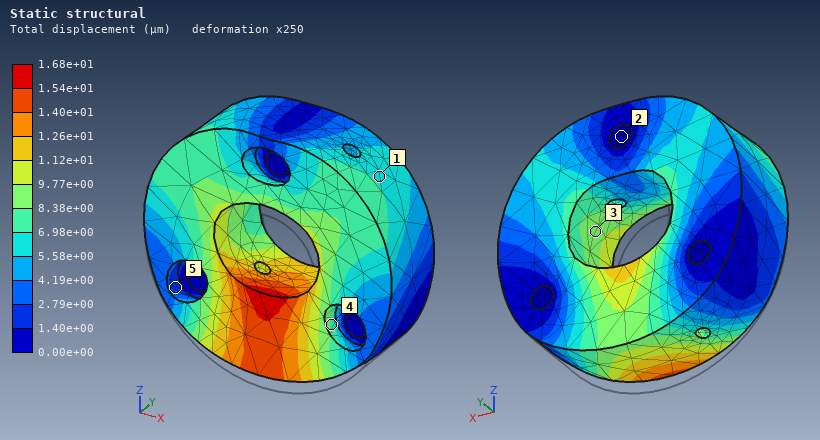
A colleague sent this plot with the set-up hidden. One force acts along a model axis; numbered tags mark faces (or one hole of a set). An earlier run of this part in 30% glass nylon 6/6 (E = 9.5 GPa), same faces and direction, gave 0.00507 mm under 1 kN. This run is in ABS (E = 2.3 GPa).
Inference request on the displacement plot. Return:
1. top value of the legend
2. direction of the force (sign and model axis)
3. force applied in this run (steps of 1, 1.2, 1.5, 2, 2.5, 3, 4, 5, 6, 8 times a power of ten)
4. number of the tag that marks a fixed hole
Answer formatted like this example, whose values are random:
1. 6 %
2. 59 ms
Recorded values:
1. 1.68e+01 µm
2. +Z
3. 800 N
4. 2
